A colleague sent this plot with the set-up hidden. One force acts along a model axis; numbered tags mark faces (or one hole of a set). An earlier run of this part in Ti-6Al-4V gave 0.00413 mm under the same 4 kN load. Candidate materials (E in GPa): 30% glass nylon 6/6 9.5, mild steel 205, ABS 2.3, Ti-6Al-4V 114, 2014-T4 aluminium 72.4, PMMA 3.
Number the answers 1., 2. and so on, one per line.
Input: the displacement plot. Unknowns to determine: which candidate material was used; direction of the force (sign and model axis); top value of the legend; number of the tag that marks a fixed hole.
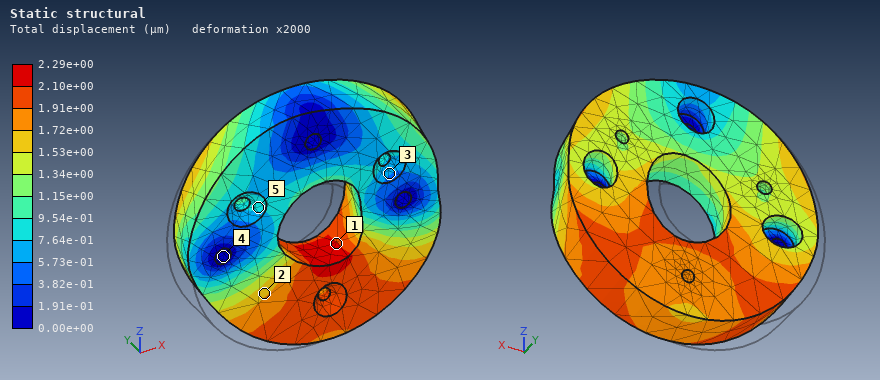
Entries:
1. mild steel
2. +X
3. 2.29e+00 µm
4. 4
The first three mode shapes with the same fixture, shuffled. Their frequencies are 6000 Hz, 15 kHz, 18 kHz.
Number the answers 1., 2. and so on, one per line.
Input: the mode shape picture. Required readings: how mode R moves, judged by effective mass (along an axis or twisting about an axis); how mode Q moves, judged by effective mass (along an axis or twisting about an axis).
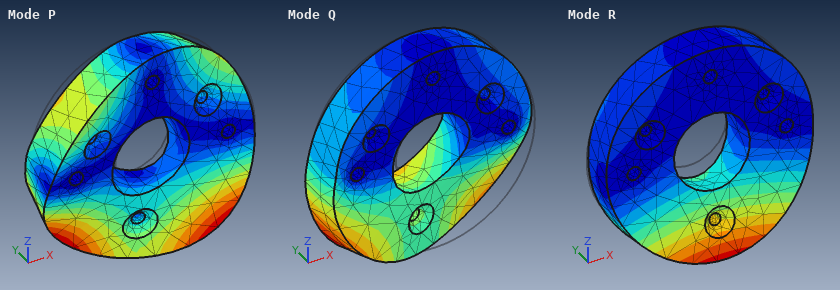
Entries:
1. along Y
2. along X
